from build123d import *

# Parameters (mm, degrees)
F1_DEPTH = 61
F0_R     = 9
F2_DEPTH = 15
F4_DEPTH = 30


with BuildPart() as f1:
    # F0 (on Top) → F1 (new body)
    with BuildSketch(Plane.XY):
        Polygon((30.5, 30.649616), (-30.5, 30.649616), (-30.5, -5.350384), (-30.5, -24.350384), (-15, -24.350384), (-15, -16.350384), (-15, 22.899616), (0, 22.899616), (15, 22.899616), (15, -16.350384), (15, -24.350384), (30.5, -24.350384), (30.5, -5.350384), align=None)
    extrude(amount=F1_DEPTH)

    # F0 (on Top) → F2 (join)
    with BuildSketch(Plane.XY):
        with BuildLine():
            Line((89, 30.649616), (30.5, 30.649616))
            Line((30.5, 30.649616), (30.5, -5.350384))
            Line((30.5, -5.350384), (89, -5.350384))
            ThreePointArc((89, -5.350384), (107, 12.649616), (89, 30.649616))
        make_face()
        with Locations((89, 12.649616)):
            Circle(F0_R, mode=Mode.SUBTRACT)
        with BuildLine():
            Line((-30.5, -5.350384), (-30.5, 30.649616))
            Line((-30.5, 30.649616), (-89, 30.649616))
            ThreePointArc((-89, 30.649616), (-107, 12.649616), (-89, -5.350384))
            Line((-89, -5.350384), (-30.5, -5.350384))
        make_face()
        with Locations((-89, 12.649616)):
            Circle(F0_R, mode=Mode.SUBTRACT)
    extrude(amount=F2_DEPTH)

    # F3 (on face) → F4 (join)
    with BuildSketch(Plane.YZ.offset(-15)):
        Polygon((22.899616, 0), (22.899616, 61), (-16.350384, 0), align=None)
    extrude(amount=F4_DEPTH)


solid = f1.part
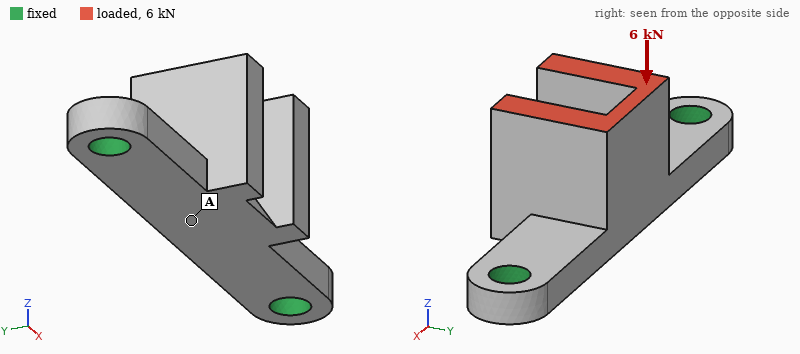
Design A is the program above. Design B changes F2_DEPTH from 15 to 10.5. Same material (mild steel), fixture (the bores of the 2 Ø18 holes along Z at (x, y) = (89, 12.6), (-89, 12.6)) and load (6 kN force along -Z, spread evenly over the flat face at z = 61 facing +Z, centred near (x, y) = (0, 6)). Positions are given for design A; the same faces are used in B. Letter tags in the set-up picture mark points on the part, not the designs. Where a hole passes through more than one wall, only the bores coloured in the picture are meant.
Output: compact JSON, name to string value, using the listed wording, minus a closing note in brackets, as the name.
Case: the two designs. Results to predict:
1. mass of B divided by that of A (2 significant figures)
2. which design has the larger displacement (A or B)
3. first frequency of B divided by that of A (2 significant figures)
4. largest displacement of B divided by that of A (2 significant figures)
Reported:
{"mass of B divided by that of A": "0.91", "which design has the larger displacement": "B", "first frequency of B divided by that of A": "0.63", "largest displacement of B divided by that of A": "2.4"}
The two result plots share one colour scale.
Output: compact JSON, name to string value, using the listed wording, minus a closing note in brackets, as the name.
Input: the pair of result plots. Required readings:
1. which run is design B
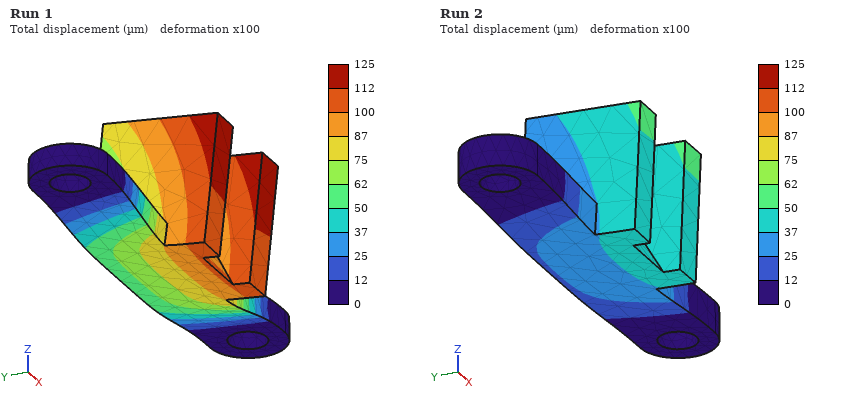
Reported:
{"which run is design B": "Run 1"}
